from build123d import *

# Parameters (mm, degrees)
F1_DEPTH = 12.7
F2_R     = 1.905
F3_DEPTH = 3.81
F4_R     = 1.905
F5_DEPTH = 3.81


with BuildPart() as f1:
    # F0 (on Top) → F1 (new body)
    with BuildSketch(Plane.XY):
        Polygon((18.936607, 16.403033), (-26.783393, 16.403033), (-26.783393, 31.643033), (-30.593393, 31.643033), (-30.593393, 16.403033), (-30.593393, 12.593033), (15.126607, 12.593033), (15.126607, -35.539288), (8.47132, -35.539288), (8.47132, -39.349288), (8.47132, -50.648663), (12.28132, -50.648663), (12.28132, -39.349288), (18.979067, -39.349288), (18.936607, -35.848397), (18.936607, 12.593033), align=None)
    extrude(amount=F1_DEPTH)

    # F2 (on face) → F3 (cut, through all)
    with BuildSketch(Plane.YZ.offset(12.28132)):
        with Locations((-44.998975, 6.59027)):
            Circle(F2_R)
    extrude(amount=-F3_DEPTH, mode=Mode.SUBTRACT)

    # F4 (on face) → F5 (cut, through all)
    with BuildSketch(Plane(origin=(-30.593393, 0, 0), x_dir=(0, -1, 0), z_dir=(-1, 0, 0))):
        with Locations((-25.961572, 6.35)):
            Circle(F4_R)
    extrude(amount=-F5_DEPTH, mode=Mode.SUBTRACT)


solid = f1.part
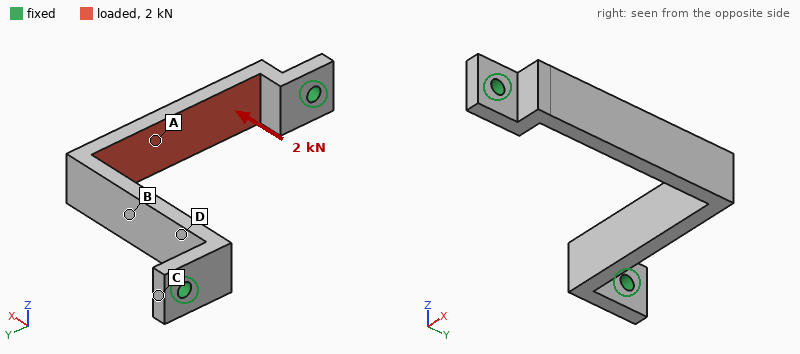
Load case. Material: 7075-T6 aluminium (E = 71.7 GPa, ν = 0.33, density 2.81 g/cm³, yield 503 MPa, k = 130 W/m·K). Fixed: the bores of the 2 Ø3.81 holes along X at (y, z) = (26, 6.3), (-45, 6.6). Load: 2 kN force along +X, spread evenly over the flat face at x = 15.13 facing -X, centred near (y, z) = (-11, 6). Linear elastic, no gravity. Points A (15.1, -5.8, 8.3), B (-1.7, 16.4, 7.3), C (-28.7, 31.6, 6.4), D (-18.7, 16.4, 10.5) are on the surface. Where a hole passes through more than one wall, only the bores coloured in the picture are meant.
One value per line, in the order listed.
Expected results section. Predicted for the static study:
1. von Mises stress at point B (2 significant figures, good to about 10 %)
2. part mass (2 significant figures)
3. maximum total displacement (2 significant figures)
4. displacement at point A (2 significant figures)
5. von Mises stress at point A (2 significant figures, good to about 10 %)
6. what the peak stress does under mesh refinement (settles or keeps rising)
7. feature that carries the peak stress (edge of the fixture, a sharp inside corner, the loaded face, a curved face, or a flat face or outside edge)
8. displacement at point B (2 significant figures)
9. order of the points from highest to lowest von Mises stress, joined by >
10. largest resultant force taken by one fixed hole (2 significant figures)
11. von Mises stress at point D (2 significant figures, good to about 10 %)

56 MPa
18 g
0.46 mm
0.42 mm
190 MPa
keeps rising
edge of the fixture
0.16 mm
A > D > B > C
1.1 kN
99 MPa
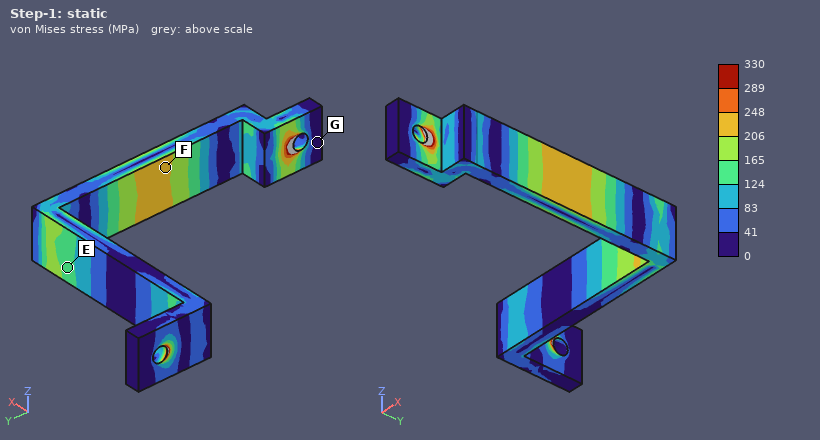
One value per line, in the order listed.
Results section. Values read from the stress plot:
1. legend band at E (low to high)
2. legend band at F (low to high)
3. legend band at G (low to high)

124 to 165 MPa
206 to 248 MPa
0 to 41 MPa
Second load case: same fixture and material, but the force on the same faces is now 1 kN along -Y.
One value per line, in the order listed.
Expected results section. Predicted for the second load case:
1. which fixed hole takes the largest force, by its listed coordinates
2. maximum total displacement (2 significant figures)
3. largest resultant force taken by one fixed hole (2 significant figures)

(-45, 6.6)
92 µm
970 N
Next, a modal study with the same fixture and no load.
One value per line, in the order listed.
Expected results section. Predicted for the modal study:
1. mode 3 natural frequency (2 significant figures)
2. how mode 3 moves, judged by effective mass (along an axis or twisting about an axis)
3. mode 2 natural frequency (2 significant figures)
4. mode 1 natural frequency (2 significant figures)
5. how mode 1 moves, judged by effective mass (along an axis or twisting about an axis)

5200 Hz
along X
4000 Hz
1900 Hz
along Z
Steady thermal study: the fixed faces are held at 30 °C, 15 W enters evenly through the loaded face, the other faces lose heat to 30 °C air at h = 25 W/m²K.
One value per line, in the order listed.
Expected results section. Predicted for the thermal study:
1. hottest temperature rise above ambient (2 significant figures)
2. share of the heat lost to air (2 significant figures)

42 K
13 %
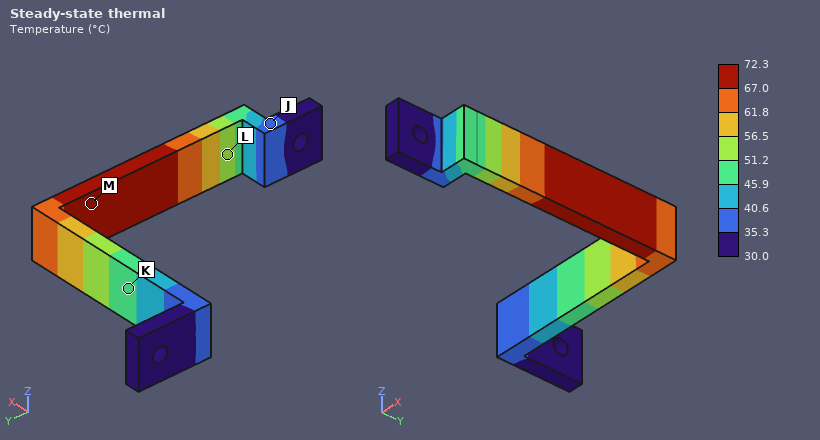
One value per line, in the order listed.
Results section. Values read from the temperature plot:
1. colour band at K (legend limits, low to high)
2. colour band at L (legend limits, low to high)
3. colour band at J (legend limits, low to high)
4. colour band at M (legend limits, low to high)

45.9 to 51.2 °C
51.2 to 56.5 °C
35.3 to 40.6 °C
67.0 to 72.3 °C
